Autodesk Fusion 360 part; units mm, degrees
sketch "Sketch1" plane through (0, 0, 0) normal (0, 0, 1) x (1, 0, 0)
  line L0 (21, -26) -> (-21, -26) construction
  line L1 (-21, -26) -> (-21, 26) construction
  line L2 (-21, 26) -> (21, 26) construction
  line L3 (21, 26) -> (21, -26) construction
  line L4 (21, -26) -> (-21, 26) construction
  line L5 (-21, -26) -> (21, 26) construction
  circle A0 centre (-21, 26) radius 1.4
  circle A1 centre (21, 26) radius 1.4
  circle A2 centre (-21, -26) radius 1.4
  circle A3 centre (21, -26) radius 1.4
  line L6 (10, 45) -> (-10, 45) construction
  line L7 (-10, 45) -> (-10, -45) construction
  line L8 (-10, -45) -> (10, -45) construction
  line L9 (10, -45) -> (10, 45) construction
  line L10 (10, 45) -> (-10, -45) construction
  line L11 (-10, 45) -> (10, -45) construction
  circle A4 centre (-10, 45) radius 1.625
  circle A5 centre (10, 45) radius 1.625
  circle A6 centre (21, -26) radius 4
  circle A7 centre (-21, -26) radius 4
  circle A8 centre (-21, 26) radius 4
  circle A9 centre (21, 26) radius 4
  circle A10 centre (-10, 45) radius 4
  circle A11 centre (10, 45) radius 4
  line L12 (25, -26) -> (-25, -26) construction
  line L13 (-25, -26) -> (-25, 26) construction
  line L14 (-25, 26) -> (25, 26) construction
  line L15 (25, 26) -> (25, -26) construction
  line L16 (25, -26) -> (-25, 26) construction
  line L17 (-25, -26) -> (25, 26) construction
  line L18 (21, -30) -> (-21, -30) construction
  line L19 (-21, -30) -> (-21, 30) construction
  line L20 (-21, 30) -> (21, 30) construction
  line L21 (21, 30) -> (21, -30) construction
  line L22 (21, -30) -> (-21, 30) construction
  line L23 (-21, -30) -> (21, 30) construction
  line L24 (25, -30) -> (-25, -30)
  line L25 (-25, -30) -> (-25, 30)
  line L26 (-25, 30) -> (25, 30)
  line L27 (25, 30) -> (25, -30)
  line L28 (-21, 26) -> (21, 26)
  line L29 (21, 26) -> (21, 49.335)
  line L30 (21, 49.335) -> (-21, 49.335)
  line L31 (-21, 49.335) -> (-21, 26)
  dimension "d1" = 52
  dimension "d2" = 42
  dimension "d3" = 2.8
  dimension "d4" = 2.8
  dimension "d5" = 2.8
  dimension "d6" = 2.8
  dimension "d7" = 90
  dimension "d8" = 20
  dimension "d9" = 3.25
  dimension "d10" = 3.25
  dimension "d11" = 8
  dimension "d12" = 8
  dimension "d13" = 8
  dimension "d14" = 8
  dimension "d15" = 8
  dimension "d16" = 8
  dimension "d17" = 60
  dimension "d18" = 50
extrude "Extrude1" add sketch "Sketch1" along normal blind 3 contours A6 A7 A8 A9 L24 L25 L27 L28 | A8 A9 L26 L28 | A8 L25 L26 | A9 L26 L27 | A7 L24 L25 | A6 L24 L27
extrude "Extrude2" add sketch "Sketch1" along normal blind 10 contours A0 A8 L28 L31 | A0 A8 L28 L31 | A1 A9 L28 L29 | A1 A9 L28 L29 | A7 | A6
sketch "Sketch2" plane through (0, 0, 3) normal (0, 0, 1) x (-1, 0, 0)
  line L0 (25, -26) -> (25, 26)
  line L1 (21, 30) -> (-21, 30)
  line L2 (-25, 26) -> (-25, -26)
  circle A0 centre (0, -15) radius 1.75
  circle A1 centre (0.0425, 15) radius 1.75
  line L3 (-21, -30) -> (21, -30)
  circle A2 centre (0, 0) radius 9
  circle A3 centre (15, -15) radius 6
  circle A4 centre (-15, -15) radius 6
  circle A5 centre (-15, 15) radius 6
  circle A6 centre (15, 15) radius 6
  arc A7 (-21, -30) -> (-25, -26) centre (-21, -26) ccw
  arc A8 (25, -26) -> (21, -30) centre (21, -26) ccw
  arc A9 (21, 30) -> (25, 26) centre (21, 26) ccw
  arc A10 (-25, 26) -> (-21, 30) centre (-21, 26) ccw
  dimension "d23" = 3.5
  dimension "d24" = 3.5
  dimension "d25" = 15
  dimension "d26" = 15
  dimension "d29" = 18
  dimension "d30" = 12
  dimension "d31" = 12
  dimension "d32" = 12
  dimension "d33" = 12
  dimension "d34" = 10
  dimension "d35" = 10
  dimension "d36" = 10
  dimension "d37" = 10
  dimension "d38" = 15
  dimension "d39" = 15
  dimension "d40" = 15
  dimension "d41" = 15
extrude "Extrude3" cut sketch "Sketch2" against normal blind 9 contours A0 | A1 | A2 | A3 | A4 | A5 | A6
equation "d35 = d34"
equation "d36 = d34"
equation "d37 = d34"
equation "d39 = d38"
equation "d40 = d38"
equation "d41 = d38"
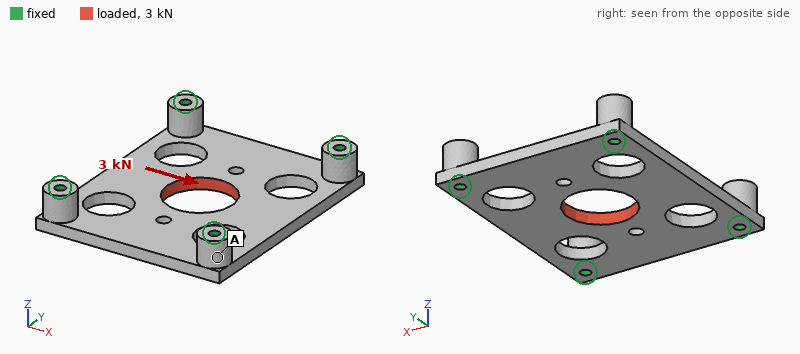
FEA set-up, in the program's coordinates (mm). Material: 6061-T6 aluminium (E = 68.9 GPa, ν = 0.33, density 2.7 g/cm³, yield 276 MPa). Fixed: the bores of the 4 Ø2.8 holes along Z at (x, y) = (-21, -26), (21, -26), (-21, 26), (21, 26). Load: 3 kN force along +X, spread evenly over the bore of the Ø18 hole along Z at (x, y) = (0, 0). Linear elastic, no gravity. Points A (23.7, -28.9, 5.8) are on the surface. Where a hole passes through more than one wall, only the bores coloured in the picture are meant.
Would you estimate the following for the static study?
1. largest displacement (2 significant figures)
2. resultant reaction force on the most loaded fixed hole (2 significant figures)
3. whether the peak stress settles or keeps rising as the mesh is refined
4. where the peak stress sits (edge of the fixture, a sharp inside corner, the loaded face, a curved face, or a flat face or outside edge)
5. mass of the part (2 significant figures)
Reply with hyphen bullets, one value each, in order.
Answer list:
- 25 µm
- 840 N
- keeps rising
- a sharp inside corner
- 22 g
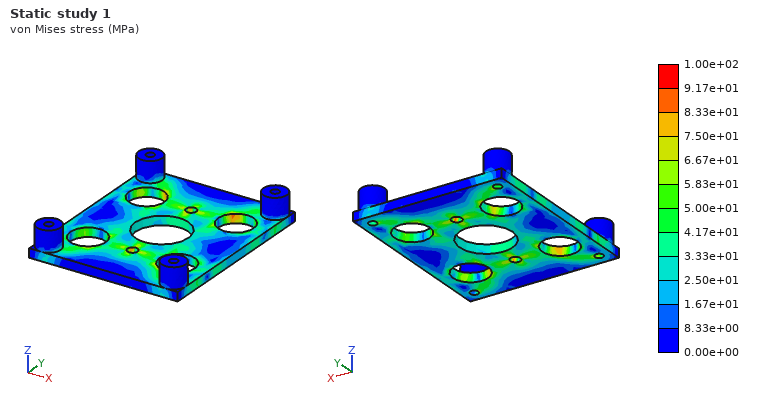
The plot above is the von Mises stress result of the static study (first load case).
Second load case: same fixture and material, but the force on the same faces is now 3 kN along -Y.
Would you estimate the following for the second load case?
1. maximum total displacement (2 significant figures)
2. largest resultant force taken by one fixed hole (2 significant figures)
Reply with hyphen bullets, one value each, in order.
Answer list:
- 20 µm
- 800 N
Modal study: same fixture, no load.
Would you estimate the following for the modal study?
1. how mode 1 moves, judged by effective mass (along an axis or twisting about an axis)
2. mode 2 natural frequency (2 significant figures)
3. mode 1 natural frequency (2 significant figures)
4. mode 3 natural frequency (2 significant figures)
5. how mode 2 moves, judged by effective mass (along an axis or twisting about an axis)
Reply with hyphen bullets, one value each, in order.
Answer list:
- along Z
- 6700 Hz
- 4800 Hz
- 8800 Hz
- twisting about Y
